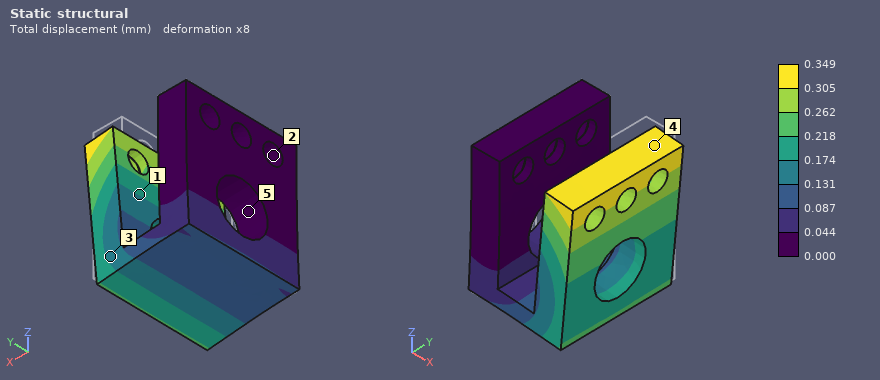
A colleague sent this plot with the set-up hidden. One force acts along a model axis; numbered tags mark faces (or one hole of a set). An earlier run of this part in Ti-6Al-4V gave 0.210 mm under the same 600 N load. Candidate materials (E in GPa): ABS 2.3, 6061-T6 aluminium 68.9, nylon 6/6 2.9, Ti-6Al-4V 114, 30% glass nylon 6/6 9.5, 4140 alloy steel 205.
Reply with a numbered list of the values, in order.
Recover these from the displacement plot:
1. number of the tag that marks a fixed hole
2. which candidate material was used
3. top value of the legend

1. 2
2. 6061-T6 aluminium
3. 0.349 mm
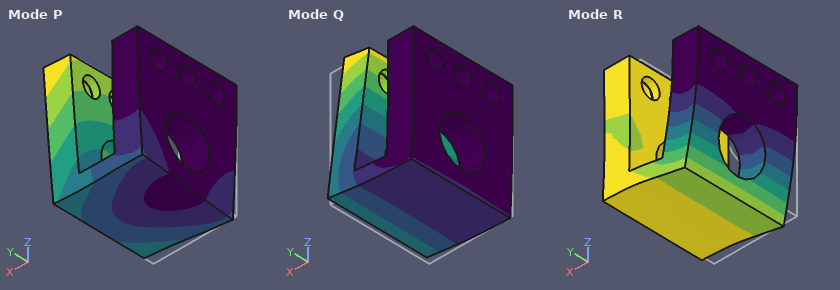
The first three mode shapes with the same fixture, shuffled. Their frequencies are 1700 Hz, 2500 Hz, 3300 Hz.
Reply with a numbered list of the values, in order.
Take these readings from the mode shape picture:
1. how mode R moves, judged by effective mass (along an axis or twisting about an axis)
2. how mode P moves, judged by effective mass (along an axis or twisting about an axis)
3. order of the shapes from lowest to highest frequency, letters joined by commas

1. along X
2. along Y
3. Q, P, R
